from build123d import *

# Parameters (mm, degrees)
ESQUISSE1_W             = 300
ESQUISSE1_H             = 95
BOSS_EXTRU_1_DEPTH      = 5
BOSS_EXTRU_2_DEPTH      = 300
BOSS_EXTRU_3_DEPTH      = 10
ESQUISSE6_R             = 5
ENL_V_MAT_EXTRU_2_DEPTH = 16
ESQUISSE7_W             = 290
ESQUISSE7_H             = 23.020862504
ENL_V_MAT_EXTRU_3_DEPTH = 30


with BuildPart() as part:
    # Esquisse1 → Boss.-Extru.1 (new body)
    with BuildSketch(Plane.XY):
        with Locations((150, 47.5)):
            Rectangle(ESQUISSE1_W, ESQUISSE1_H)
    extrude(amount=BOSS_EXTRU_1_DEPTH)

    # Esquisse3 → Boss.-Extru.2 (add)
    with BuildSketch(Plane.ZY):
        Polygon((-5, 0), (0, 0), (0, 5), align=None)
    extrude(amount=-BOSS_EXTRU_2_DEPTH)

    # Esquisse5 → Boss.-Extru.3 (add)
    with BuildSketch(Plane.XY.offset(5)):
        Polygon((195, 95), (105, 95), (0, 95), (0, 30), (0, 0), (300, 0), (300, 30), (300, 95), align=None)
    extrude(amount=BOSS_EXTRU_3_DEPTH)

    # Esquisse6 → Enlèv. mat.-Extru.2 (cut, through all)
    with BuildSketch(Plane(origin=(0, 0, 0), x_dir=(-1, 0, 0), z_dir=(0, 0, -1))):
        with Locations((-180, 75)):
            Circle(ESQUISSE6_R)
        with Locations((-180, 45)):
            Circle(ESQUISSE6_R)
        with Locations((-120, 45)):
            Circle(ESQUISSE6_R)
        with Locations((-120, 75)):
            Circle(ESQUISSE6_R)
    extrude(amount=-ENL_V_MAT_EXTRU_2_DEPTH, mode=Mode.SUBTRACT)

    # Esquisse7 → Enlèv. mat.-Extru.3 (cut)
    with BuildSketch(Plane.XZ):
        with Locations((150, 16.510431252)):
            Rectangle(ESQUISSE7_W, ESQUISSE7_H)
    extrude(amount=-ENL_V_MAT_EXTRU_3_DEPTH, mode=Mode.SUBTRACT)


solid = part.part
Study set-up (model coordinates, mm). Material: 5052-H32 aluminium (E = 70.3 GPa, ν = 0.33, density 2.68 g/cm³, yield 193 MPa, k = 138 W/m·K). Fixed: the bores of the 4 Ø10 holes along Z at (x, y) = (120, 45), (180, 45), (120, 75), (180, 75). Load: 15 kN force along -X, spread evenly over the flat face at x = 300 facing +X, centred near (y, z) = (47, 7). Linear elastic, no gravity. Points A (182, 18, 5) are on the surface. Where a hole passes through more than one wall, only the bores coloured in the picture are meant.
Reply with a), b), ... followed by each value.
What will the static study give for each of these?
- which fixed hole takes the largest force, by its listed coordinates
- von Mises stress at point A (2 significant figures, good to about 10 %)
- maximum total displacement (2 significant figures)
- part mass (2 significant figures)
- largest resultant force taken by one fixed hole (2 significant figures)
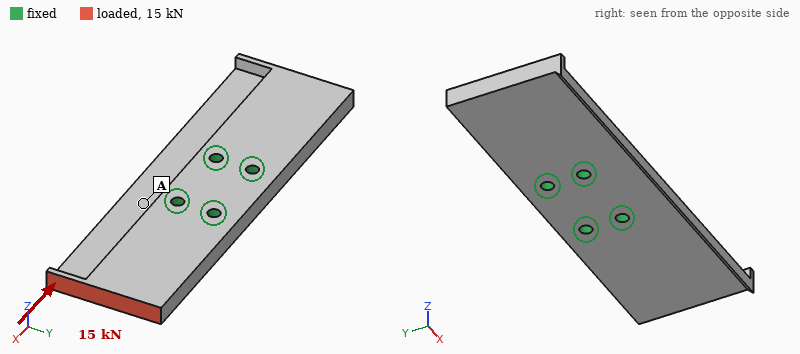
a) (180, 45)
b) 14 MPa
c) 0.22 mm
d) 910 g
e) 9.5 kN
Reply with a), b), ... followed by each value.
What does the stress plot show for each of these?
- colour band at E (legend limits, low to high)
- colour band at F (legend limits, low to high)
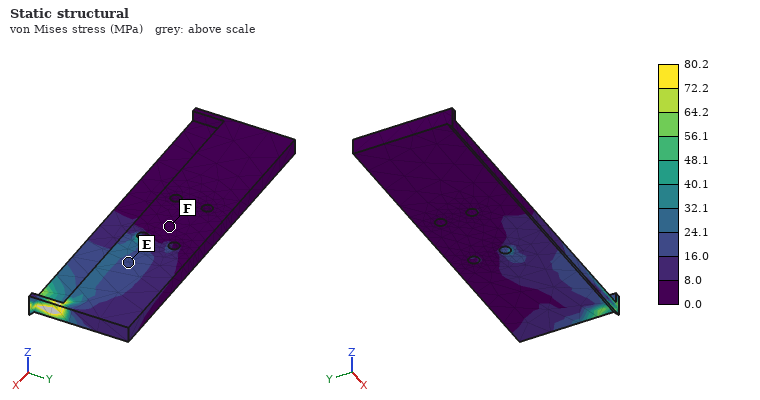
a) 16.0 to 24.1 MPa
b) 0.0 to 8.0 MPa
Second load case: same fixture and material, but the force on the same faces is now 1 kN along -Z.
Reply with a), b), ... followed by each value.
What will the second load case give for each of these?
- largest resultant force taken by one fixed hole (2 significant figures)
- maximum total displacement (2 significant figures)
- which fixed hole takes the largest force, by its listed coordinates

a) 1.5 kN
b) 0.46 mm
c) (180, 45)
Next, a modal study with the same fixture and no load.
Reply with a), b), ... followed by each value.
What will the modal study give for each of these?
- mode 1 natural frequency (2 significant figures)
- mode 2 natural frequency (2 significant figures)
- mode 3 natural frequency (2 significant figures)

a) 830 Hz
b) 830 Hz
c) 2100 Hz
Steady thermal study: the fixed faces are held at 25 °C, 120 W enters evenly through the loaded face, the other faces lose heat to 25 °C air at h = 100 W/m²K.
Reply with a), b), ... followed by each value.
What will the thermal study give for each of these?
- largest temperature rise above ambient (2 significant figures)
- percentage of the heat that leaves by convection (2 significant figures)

a) 70 K
b) 58 %
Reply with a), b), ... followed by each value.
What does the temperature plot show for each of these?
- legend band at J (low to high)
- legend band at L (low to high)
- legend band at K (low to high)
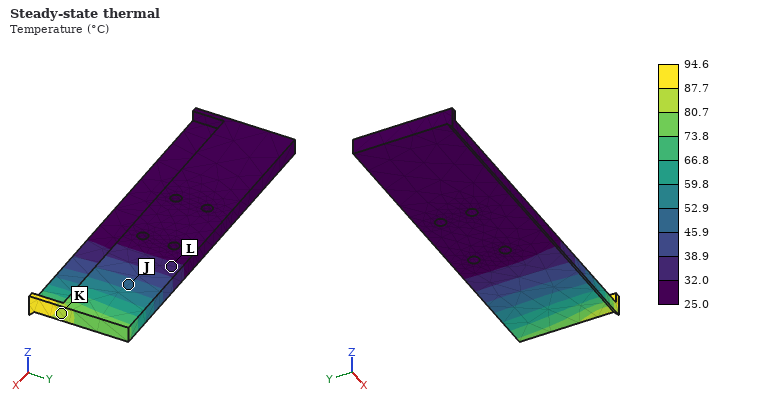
a) 45.9 to 52.9 °C
b) 32.0 to 38.9 °C
c) 80.7 to 87.7 °C
